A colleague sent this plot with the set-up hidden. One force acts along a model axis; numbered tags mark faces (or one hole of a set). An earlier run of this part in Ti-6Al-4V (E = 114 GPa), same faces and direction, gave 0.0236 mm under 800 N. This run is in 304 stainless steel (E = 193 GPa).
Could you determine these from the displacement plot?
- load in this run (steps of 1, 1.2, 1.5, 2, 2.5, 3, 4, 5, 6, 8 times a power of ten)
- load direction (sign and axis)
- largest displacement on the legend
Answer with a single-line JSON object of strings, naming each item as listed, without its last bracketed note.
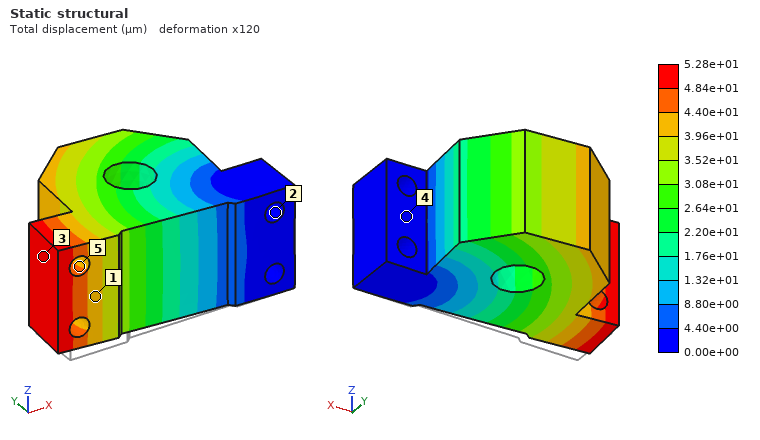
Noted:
{"load in this run": "3 kN", "load direction": "+Y", "largest displacement on the legend": "5.28e+01 µm"}
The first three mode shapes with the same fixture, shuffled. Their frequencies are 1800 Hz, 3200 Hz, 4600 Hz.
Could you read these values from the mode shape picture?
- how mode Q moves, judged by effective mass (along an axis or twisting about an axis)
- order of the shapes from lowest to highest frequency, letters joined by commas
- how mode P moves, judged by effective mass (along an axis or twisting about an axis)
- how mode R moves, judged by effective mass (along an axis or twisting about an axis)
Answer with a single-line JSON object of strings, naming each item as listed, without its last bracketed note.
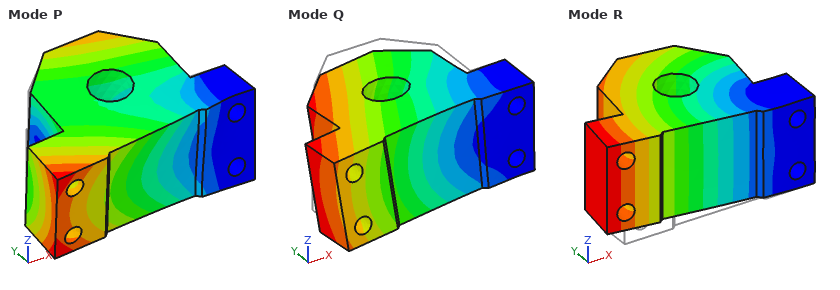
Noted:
{"how mode Q moves, judged by effective mass": "along Z", "order of the shapes from lowest to highest frequency, letters joined by commas": "R, Q, P", "how mode P moves, judged by effective mass": "twisting about X", "how mode R moves, judged by effective mass": "along Y"}
